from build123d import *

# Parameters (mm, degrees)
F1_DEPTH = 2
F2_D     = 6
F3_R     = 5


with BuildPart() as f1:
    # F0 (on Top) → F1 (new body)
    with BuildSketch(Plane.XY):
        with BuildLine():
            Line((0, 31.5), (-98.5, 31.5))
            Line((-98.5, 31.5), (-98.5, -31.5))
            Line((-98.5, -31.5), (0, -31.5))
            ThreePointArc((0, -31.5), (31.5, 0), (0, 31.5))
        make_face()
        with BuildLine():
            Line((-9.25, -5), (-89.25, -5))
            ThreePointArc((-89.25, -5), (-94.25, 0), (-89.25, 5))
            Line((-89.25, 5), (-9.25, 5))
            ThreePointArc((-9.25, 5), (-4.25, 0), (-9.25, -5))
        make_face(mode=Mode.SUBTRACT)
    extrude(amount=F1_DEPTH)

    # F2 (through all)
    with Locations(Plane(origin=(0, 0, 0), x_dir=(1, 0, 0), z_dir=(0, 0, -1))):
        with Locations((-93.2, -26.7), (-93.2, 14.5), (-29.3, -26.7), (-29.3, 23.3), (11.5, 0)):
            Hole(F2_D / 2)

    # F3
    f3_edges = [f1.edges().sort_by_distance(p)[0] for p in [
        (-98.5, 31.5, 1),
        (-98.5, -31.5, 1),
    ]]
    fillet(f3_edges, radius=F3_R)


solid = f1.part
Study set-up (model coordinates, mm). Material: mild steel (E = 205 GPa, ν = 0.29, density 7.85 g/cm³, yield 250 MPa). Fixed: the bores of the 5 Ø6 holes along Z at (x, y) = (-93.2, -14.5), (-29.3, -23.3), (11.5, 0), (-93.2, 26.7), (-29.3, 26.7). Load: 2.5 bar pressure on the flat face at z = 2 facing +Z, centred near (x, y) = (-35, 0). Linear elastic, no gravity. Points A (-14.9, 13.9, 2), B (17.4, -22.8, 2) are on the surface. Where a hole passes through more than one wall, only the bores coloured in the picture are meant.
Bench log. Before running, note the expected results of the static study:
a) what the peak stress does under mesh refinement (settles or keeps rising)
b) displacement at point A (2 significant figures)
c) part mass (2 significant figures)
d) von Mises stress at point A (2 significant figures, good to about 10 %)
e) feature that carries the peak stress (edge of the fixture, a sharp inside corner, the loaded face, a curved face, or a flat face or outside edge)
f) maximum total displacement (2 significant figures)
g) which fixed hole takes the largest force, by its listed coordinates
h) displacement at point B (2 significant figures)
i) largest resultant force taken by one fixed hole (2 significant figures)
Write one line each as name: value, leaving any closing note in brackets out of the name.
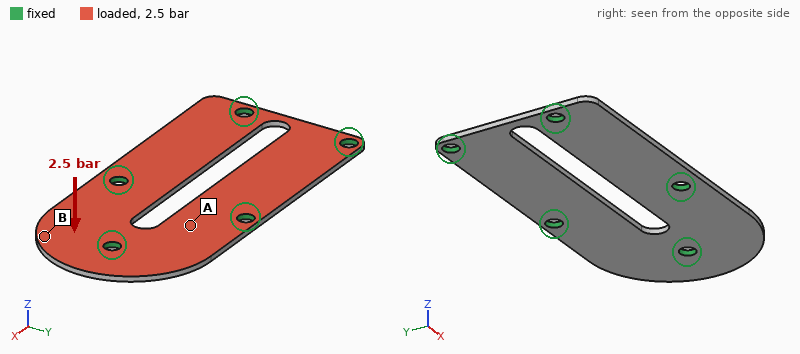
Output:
what the peak stress does under mesh refinement: keeps rising
displacement at point A: 0.021 mm
part mass: 110 g
von Mises stress at point A: 46 MPa
feature that carries the peak stress: edge of the fixture
maximum total displacement: 0.13 mm
which fixed hole takes the largest force, by its listed coordinates: (11.5, 0)
displacement at point B: 0.058 mm
largest resultant force taken by one fixed hole: 460 N
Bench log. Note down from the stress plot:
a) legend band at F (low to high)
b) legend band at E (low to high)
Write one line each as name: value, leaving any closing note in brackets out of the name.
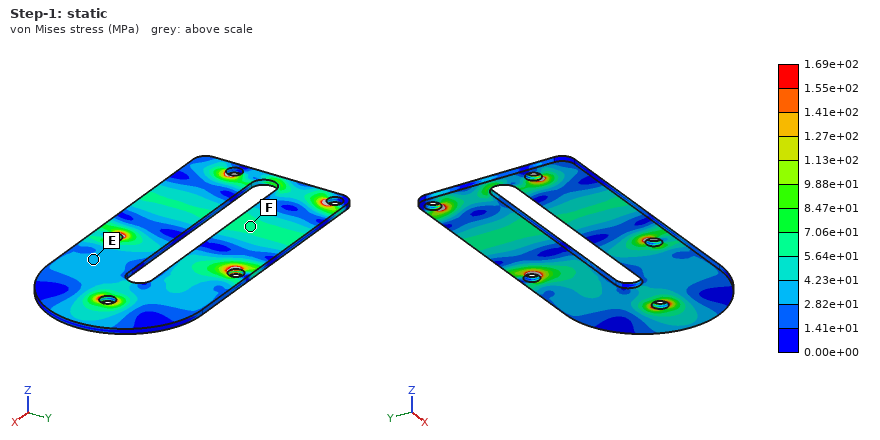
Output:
legend band at F: 5.64e+01 to 7.06e+01 MPa
legend band at E: 2.82e+01 to 4.23e+01 MPa
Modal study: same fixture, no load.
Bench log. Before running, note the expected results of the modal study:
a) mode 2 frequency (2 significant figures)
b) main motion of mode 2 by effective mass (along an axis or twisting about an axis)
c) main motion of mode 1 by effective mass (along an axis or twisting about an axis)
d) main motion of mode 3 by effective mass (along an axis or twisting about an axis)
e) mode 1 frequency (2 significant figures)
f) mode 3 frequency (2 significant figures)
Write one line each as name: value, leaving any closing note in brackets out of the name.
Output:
mode 2 frequency: 2600 Hz
main motion of mode 2 by effective mass: along Z
main motion of mode 1 by effective mass: along Z
main motion of mode 3 by effective mass: twisting about X
mode 1 frequency: 2200 Hz
mode 3 frequency: 2800 Hz
